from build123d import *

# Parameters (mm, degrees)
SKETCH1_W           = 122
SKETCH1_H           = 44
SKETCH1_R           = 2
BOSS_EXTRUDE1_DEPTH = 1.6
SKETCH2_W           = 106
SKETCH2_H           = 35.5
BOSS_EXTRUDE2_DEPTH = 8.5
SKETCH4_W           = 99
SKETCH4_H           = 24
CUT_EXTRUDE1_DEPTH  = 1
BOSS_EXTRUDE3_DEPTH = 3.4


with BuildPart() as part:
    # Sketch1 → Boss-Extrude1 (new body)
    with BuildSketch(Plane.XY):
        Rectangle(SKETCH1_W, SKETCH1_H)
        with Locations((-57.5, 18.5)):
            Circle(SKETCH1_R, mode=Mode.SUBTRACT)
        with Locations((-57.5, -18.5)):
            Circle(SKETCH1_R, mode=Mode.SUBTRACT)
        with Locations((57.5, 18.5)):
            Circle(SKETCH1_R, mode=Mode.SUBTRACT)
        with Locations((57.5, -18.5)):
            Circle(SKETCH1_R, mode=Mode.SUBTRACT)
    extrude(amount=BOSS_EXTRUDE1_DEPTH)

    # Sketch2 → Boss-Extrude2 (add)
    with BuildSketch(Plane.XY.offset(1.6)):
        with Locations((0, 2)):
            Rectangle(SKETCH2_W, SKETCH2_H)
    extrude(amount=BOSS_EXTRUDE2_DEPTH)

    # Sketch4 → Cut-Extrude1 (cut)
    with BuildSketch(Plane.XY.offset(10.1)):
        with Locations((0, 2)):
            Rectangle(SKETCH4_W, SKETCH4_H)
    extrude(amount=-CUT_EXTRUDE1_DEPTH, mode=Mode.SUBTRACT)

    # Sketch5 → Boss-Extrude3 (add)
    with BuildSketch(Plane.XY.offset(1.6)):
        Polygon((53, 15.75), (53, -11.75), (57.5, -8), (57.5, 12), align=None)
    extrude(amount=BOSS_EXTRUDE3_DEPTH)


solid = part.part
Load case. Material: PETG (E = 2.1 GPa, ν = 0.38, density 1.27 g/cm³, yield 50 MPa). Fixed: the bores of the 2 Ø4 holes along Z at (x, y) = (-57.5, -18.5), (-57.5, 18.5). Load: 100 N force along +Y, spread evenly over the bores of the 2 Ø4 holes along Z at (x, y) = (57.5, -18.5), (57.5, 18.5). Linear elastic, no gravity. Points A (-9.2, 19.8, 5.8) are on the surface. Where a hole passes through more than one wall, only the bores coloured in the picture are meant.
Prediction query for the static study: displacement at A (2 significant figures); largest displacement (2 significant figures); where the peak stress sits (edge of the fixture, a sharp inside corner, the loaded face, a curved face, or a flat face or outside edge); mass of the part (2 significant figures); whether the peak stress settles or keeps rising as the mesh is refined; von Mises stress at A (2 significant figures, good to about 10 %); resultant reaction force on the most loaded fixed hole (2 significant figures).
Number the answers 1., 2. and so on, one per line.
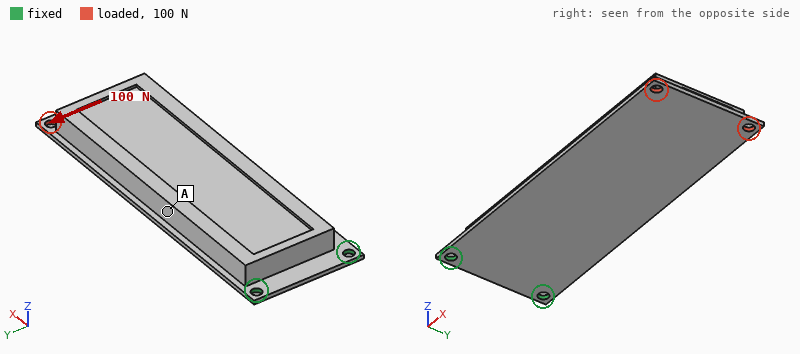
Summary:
1. 0.40 mm
2. 1.5 mm
3. edge of the fixture
4. 49 g
5. keeps rising
6. 2.8 MPa
7. 320 N
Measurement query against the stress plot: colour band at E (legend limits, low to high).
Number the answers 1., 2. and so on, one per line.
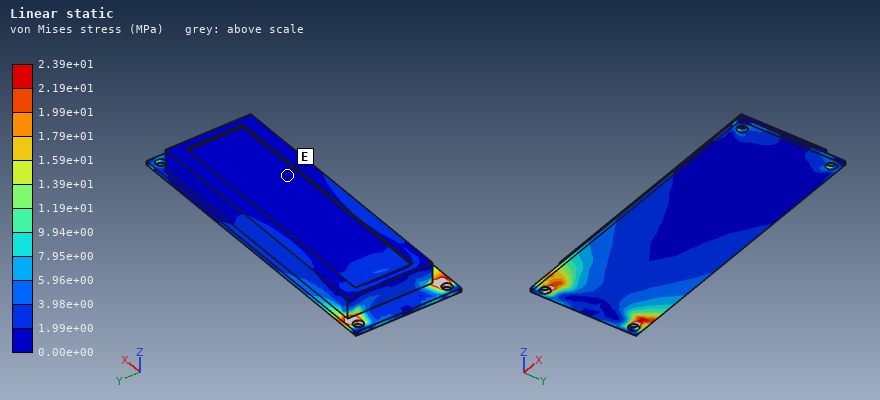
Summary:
1. 0.00e+00 to 1.99e+00 MPa
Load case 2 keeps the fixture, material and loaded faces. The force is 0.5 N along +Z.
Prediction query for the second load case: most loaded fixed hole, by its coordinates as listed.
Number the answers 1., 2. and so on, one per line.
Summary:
1. (-57.5, -18.5)
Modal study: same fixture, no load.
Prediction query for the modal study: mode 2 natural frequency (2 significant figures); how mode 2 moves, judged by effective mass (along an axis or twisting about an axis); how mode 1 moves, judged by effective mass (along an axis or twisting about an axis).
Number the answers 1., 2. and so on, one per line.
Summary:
1. 390 Hz
2. along Y
3. along Z
